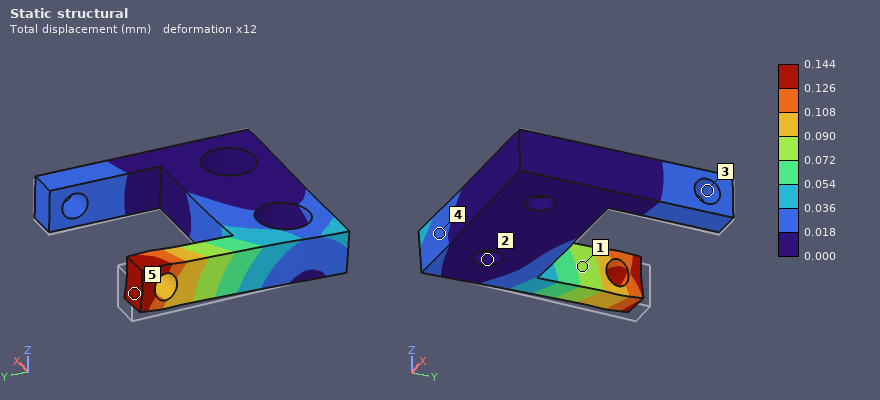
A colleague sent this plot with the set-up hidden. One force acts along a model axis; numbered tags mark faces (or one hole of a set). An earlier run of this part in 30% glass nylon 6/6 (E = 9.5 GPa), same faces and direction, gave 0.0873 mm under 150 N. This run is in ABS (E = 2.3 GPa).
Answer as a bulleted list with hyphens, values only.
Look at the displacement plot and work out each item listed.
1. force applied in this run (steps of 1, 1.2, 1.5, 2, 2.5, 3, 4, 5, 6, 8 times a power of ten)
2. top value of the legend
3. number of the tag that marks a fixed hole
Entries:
- 60 N
- 0.144 mm
- 2
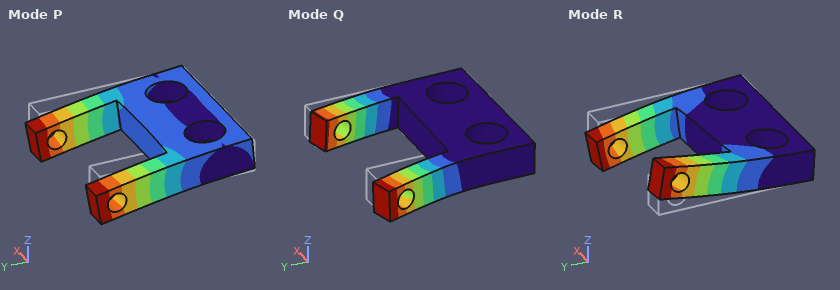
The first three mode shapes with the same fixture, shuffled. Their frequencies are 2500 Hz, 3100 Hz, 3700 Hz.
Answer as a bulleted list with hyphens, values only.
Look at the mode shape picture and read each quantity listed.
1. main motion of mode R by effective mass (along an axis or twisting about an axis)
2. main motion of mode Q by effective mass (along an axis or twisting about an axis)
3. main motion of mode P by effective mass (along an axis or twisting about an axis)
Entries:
- twisting about Y
- along X
- along Z
